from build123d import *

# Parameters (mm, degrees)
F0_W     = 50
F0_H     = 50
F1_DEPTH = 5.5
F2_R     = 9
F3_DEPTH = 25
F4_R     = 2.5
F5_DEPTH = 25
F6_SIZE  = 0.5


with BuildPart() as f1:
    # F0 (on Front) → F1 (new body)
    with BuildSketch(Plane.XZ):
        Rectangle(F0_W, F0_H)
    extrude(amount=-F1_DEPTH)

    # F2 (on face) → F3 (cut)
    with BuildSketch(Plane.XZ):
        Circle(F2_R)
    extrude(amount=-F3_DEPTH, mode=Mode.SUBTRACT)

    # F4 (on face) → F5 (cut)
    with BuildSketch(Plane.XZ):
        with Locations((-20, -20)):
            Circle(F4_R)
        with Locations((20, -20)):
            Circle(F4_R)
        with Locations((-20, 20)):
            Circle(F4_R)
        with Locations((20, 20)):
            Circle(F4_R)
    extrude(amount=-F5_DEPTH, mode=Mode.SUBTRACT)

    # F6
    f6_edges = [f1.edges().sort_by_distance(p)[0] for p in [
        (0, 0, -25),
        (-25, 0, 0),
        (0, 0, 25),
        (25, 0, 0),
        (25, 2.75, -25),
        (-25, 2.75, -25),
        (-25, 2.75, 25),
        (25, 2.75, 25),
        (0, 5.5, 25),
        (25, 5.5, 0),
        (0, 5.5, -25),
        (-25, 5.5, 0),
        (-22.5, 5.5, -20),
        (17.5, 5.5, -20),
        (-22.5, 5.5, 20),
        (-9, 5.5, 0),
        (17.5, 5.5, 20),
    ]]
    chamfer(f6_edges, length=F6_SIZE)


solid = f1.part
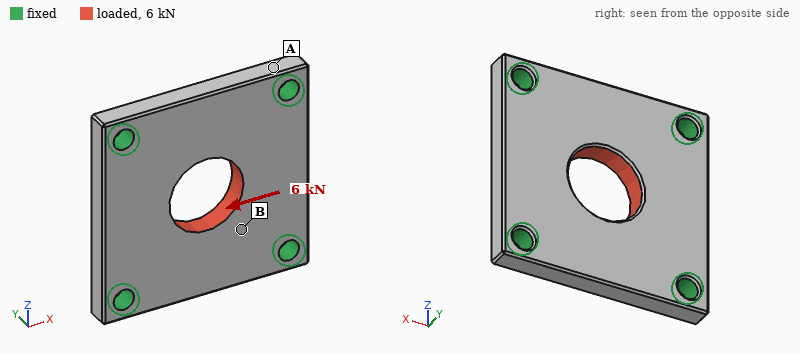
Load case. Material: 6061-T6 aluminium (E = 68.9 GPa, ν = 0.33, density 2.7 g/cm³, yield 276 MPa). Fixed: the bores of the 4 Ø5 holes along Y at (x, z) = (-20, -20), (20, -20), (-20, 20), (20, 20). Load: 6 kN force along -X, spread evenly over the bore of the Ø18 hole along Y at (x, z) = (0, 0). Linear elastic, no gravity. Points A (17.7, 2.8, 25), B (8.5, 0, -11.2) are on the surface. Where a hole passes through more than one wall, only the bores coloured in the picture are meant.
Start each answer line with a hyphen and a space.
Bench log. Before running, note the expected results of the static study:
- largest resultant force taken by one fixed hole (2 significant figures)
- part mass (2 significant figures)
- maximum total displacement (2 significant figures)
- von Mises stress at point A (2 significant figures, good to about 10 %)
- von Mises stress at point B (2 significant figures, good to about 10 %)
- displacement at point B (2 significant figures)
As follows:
- 1.7 kN
- 32 g
- 10 µm
- 9.3 MPa
- 20 MPa
- 5.5 µm
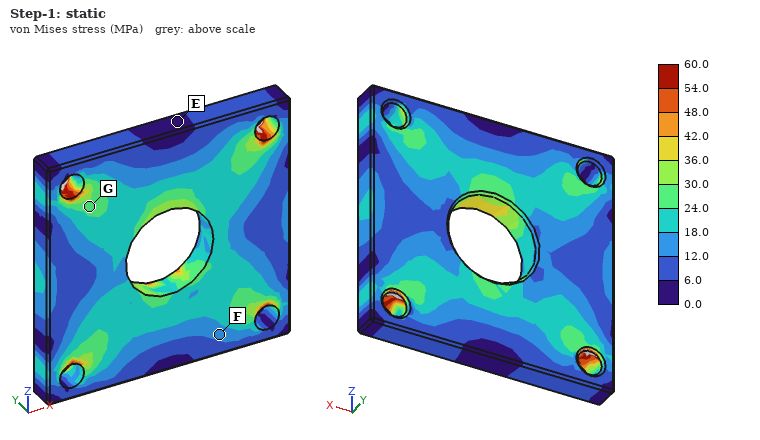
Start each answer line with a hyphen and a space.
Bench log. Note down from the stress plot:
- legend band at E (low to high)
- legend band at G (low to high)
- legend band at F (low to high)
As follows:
- 0.0 to 6.0 MPa
- 24.0 to 30.0 MPa
- 12.0 to 18.0 MPa
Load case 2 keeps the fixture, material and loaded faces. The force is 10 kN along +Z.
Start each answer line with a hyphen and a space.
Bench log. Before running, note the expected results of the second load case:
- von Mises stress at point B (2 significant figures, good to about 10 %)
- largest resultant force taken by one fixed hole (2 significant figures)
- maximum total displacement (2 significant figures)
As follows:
- 36 MPa
- 2.8 kN
- 17 µm
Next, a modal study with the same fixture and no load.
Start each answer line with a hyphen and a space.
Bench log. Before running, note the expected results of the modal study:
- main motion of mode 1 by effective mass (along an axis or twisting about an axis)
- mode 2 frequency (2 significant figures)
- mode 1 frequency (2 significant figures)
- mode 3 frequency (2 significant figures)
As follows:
- along Y
- 18 kHz
- 13 kHz
- 18 kHz
